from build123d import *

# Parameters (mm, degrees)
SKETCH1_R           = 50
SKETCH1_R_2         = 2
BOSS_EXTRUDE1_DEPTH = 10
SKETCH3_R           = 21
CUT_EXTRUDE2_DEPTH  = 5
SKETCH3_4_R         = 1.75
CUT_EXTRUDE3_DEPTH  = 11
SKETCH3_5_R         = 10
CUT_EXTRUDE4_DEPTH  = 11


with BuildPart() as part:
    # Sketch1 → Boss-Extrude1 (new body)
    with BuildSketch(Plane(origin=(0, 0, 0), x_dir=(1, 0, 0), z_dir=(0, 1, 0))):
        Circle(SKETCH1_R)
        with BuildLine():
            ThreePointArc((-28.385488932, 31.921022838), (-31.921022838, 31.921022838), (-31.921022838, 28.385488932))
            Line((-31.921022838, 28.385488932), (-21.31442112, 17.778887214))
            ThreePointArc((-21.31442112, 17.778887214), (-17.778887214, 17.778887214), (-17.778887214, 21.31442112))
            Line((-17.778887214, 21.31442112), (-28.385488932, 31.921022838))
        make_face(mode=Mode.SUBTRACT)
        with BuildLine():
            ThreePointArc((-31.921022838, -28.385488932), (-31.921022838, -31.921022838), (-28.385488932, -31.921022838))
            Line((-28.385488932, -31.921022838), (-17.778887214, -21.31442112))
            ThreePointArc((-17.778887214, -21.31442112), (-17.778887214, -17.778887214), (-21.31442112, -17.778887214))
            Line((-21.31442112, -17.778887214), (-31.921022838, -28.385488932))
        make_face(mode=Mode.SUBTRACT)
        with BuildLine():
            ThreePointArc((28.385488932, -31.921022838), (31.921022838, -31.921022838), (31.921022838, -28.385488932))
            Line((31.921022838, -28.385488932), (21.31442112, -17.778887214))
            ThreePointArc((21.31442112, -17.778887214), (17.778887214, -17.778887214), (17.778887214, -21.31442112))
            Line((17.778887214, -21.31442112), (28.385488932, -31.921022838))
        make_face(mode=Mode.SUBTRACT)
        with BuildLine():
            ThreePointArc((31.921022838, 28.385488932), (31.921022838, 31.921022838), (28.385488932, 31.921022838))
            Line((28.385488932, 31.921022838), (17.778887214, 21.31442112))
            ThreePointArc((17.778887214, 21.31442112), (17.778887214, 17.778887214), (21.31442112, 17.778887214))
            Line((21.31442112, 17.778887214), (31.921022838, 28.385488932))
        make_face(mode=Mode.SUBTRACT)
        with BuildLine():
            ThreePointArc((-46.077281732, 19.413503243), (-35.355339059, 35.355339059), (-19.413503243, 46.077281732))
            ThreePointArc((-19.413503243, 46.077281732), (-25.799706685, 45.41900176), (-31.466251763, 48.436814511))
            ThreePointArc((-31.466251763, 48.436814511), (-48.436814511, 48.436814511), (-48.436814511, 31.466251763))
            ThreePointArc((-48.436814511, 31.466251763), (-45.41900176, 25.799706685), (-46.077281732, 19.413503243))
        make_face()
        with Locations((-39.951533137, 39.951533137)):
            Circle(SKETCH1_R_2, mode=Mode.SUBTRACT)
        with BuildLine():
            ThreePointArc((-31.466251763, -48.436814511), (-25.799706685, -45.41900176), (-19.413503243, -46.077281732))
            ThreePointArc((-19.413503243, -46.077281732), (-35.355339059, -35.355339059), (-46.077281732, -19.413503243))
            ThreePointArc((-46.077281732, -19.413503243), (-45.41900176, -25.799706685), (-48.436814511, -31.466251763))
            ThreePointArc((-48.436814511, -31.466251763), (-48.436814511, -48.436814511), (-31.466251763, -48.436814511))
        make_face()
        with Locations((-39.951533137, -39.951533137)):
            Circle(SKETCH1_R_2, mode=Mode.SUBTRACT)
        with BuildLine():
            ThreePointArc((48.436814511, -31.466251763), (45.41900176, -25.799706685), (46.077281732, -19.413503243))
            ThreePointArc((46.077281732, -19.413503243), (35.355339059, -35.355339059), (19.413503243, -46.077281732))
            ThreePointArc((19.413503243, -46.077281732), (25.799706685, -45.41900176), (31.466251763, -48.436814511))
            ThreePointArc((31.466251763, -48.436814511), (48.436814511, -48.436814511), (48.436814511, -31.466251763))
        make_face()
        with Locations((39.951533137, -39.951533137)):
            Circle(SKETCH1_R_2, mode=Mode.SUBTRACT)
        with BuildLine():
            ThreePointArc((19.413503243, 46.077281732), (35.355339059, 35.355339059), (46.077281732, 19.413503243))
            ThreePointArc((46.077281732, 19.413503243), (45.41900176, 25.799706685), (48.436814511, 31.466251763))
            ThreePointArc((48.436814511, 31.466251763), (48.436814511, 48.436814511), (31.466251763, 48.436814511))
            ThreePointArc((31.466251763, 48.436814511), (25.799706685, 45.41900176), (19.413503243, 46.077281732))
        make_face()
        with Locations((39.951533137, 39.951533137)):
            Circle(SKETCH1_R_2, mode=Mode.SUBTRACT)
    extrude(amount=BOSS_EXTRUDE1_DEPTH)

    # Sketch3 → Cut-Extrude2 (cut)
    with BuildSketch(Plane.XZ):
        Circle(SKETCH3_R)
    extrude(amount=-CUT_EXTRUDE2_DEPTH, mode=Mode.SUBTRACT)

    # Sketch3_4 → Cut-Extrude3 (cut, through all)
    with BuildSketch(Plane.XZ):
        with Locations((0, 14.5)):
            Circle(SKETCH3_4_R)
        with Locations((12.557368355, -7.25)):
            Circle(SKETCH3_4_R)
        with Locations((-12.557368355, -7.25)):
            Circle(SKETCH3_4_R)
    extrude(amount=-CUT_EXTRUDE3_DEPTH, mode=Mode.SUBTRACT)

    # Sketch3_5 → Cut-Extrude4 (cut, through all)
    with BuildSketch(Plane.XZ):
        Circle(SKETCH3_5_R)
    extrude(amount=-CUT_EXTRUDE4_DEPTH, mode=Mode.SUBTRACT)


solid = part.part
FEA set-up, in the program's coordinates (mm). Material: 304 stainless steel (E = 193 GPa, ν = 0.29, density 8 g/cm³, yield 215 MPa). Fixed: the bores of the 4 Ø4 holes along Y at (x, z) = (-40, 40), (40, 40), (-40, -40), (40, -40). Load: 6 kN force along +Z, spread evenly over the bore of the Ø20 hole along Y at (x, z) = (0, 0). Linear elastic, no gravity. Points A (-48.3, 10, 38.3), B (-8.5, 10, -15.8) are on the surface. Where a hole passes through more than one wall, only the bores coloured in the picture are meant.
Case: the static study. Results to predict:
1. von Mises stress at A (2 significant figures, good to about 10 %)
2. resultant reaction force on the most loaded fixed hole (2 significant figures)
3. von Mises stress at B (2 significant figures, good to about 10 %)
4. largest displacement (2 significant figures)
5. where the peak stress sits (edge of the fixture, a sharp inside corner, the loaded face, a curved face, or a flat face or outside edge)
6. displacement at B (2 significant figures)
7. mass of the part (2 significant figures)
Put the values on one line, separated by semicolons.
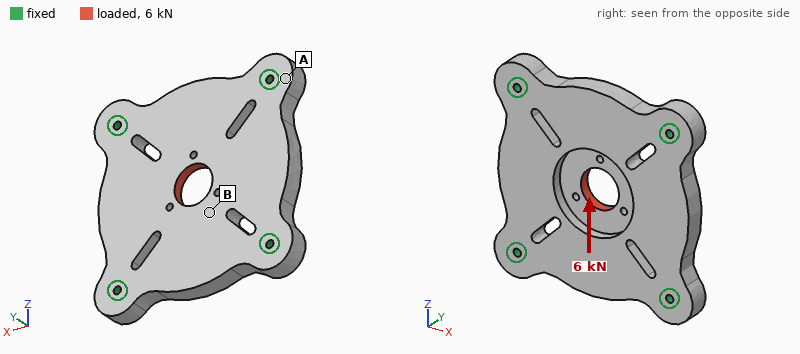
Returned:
4.0 MPa; 1.7 kN; 15 MPa; 4.5 µm; a curved face; 3.2 µm; 660 g
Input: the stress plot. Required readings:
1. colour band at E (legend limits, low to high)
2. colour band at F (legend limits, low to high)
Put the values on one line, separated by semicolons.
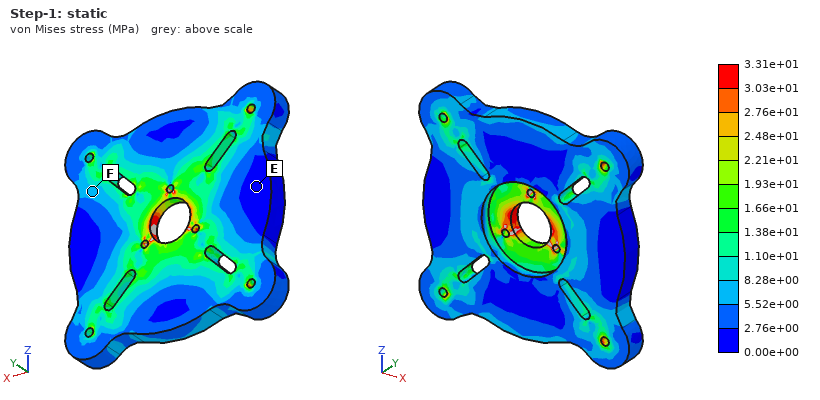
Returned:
0.00e+00 to 2.76e+00 MPa; 5.52e+00 to 8.28e+00 MPa
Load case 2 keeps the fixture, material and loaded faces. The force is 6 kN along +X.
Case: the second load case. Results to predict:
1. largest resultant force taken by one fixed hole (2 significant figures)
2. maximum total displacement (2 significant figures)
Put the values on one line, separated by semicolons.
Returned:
1.7 kN; 4.3 µm
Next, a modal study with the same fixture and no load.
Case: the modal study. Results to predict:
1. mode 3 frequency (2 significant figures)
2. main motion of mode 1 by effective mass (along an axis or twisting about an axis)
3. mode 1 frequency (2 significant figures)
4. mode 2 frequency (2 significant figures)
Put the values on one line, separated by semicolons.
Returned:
6900 Hz; along Y; 4600 Hz; 6900 Hz
